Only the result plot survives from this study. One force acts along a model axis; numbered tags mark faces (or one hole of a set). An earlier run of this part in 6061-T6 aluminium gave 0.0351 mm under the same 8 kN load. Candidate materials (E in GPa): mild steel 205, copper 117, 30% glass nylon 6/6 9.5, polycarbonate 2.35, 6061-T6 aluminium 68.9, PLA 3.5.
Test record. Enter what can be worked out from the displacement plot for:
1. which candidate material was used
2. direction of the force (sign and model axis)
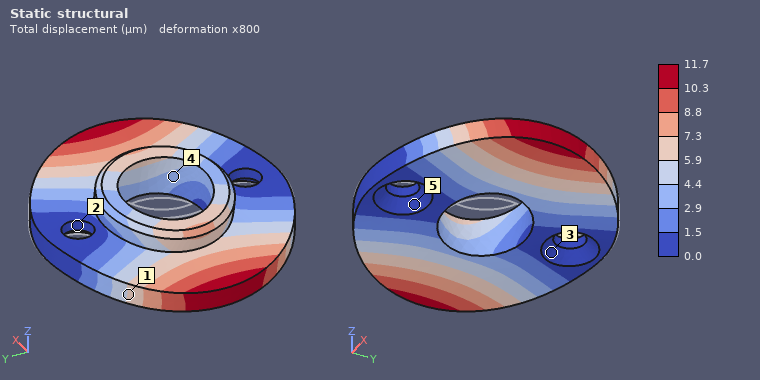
mild steel
-X
